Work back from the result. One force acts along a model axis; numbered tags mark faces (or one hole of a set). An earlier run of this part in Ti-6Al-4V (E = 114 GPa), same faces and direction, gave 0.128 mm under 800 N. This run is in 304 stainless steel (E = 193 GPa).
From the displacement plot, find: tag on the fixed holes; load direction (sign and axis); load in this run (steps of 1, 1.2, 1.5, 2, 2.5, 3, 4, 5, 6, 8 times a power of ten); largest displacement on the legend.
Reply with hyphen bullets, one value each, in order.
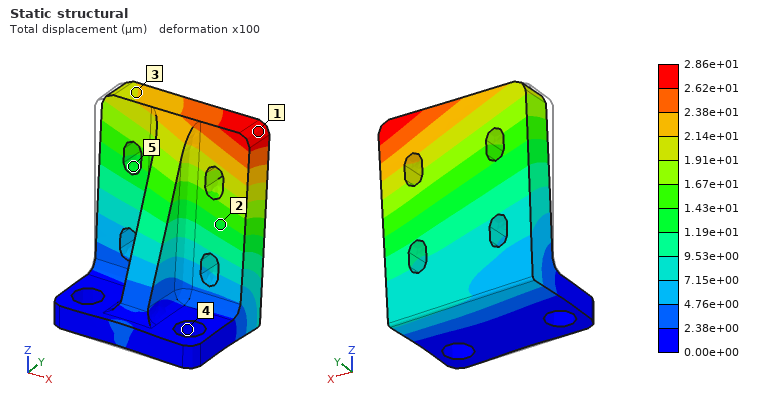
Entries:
- 4
- +Y
- 300 N
- 2.86e+01 µm
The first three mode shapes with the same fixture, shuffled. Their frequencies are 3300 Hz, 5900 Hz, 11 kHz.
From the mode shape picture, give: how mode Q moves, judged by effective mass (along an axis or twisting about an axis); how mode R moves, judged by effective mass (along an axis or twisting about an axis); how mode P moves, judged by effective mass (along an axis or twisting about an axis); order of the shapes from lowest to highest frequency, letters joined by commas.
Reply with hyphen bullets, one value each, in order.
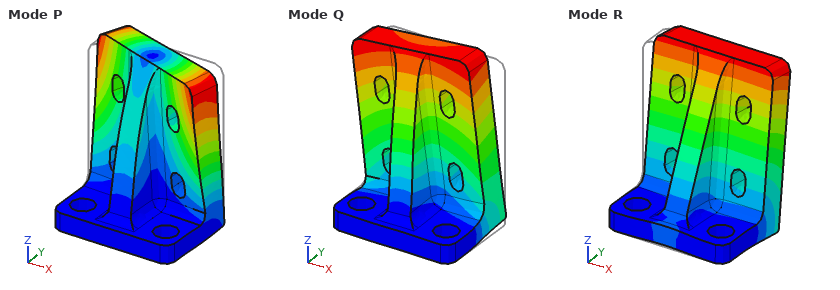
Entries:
- along X
- along Y
- twisting about Z
- R, Q, P
